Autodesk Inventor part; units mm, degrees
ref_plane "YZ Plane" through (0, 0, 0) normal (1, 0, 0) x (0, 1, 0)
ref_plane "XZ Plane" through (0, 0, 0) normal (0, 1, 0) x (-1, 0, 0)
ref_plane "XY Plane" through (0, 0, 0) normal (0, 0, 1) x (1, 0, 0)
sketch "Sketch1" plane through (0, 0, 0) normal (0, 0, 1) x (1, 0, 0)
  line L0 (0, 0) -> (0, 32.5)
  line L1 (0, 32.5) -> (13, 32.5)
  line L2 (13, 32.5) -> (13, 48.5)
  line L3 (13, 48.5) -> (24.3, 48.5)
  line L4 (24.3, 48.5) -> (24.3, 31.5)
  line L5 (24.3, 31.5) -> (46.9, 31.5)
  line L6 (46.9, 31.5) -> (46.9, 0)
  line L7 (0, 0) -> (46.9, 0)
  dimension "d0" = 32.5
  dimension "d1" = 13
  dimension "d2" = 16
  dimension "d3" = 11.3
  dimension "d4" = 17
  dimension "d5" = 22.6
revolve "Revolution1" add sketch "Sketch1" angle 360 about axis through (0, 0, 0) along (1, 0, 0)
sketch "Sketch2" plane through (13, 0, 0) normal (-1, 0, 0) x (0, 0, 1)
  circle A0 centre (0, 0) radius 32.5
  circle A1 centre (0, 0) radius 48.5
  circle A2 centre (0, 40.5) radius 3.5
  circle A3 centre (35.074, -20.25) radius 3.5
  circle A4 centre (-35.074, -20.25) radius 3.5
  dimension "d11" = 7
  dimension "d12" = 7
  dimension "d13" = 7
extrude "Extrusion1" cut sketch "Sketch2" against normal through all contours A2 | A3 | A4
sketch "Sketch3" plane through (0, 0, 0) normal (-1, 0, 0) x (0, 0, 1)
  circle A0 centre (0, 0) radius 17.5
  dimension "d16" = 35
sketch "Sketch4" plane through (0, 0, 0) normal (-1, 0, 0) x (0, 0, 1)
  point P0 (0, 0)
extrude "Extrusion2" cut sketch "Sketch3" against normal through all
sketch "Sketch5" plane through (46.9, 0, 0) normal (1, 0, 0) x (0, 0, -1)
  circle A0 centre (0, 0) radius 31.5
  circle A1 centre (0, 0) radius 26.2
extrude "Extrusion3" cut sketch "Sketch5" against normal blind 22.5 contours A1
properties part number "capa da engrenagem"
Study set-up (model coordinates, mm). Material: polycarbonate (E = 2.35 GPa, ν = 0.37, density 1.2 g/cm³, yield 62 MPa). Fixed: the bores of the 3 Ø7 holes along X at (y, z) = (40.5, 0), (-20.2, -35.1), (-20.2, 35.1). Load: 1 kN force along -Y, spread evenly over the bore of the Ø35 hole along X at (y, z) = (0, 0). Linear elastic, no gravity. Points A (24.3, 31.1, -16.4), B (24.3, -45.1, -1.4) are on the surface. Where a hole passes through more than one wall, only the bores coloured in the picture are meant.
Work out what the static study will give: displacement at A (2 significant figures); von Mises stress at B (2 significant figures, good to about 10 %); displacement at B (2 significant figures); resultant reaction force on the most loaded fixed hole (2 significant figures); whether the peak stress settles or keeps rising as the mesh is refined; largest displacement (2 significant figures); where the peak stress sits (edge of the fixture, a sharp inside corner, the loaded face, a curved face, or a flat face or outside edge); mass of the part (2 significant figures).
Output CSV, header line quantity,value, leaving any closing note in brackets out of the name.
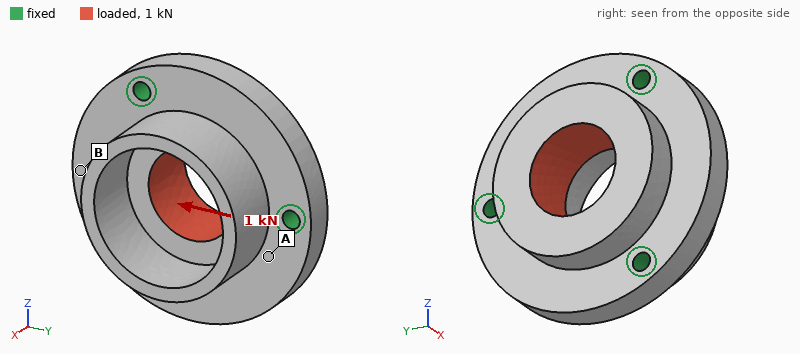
quantity,value
displacement at A,10.0 µm
von Mises stress at B,0.82 MPa
displacement at B,21 µm
resultant reaction force on the most loaded fixed hole,340 N
whether the peak stress settles or keeps rising as the mesh is refined,keeps rising
largest displacement,33 µm
where the peak stress sits,edge of the fixture
mass of the part,150 g
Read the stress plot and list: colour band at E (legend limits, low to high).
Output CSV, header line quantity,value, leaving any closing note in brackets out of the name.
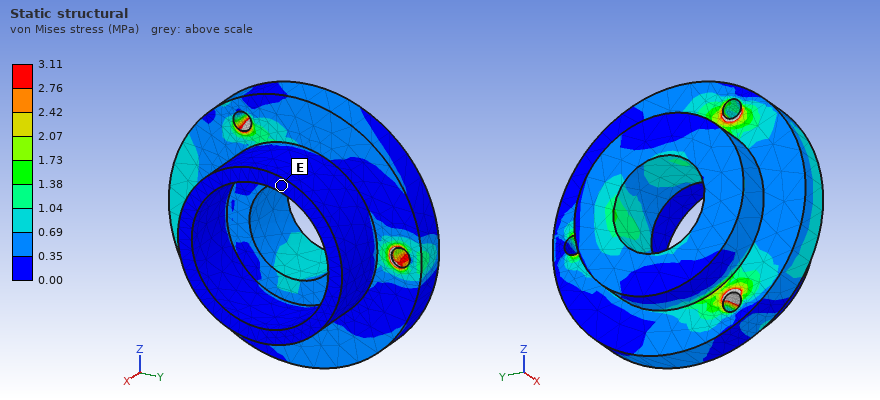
quantity,value
colour band at E,0.00 to 0.35 MPa
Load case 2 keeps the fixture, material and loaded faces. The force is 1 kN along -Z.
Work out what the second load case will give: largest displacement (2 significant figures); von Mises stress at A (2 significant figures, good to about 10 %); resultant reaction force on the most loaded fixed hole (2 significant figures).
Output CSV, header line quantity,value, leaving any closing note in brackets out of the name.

quantity,value
largest displacement,29 µm
von Mises stress at A,0.70 MPa
resultant reaction force on the most loaded fixed hole,350 N
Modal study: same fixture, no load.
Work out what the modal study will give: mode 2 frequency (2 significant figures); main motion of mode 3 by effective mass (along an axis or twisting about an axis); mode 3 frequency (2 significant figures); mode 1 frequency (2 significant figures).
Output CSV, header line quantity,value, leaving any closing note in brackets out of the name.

quantity,value
mode 2 frequency,2000 Hz
main motion of mode 3 by effective mass,along X
mode 3 frequency,2500 Hz
mode 1 frequency,2000 Hz
